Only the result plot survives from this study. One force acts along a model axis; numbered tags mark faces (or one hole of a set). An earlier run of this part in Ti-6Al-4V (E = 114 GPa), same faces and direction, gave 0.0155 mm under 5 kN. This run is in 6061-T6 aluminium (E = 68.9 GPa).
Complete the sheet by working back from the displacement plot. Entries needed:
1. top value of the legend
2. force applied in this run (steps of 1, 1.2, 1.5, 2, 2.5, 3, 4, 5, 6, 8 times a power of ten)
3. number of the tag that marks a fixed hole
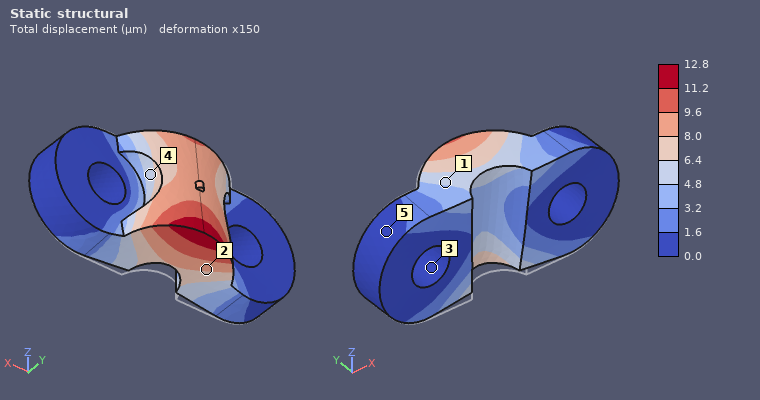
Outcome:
12.8 µm
2.5 kN
3
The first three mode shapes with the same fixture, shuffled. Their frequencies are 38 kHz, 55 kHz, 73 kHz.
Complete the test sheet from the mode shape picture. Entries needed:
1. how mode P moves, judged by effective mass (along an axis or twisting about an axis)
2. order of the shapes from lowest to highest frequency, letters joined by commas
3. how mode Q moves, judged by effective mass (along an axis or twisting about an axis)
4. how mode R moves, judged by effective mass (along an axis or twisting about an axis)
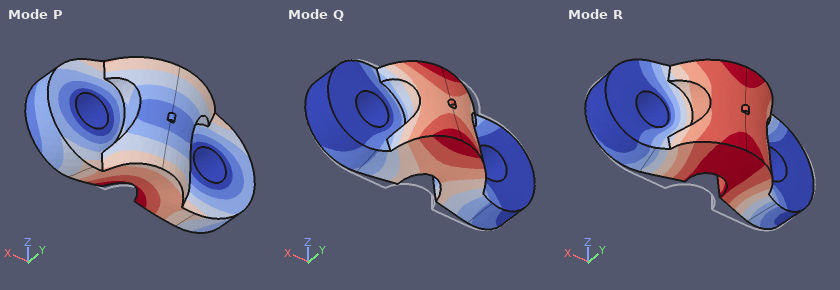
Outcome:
along Z
Q, R, P
along Z
along Y
